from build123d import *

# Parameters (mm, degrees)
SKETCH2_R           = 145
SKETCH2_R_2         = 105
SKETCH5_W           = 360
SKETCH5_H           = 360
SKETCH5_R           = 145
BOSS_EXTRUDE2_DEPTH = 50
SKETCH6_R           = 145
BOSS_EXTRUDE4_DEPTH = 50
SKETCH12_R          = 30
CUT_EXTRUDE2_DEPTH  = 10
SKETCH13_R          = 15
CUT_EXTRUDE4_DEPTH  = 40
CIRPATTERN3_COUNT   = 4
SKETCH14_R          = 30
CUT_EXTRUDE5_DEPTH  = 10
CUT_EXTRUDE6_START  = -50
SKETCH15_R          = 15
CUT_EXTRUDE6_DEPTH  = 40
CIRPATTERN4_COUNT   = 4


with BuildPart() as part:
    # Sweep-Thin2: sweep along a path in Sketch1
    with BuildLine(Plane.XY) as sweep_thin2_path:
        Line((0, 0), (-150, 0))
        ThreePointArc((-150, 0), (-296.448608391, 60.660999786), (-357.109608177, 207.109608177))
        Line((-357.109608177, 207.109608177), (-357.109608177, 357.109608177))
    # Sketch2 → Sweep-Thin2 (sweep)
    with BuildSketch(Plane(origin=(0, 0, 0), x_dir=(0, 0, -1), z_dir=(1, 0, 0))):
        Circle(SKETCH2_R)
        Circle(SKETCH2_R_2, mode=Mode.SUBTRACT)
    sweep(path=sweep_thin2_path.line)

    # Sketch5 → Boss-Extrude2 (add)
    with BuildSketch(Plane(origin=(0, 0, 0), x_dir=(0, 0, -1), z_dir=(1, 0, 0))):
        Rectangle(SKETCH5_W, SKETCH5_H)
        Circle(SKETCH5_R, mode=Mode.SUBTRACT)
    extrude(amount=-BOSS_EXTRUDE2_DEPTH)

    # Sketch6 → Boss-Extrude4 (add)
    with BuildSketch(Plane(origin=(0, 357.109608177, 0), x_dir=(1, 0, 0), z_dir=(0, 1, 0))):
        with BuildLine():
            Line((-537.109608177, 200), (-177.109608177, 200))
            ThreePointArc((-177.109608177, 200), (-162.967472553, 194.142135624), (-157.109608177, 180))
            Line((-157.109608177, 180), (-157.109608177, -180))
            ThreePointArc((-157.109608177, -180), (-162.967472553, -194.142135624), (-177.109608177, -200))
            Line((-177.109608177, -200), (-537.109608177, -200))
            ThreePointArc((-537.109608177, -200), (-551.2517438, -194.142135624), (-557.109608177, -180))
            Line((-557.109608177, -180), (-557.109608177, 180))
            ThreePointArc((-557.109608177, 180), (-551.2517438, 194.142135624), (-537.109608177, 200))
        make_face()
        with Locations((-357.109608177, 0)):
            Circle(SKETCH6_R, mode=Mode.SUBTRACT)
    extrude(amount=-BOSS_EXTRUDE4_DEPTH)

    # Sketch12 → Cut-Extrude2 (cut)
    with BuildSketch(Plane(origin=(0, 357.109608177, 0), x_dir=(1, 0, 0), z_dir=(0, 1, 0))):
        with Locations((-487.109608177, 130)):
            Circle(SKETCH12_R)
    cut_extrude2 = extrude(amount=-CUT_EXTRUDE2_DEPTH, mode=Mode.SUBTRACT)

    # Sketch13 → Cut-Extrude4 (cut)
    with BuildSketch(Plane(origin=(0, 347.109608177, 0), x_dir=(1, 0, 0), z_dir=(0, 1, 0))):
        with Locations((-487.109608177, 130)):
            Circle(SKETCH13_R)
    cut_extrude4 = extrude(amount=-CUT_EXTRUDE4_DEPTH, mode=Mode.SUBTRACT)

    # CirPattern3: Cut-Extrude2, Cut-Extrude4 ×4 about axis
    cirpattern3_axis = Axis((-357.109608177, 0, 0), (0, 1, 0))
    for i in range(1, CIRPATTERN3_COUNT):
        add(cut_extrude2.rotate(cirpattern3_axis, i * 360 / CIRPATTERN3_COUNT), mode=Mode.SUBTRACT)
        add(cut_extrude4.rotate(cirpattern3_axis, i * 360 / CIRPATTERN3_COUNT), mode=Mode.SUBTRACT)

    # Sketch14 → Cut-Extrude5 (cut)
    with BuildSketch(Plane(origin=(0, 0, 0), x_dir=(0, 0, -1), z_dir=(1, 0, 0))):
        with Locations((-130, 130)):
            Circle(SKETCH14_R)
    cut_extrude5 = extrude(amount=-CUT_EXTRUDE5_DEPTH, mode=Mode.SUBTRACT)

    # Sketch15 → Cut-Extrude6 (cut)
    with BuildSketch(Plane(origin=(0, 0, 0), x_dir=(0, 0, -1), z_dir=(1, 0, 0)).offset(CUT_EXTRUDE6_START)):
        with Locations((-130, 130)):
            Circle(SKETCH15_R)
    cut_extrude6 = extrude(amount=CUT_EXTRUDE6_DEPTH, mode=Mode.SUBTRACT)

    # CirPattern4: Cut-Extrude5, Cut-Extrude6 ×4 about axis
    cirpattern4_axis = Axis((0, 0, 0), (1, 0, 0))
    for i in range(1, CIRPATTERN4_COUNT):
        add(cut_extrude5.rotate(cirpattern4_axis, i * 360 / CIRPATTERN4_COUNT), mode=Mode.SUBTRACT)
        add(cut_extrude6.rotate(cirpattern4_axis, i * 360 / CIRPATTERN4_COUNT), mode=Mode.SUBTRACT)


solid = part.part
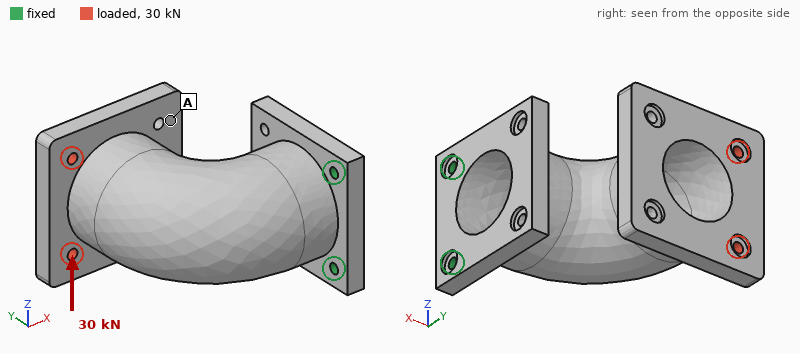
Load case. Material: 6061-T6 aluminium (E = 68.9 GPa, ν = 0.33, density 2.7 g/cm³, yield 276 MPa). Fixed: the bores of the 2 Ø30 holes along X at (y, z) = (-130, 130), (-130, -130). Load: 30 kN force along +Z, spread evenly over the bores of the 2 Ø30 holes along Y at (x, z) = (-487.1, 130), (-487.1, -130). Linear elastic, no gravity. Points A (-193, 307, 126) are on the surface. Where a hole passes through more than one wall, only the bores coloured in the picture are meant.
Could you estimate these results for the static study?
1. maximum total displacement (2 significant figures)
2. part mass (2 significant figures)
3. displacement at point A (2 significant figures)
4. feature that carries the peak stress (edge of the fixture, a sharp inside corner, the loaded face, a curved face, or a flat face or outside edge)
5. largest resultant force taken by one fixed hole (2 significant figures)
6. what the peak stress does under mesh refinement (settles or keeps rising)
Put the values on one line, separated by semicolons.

0.61 mm; 73 kg; 0.29 mm; edge of the fixture; 76 kN; keeps rising
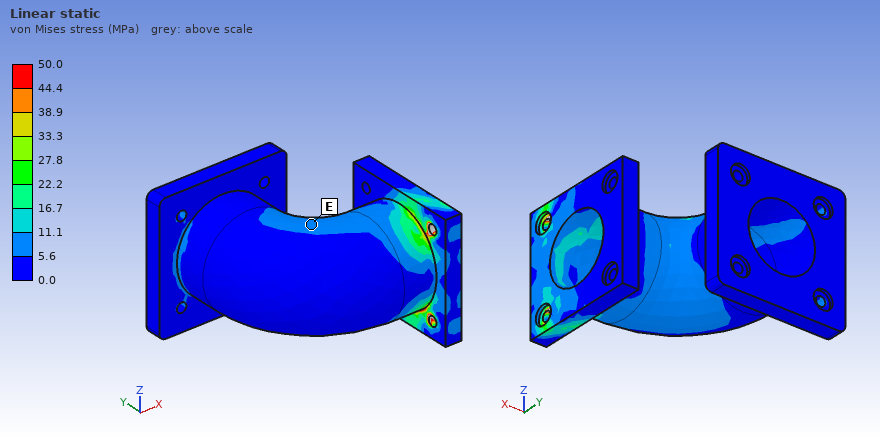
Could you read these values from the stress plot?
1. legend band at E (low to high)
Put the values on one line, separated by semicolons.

5.6 to 11.1 MPa
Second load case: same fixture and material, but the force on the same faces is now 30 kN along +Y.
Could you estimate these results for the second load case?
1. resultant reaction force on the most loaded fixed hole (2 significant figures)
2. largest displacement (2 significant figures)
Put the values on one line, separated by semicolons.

15 kN; 3.9 mm
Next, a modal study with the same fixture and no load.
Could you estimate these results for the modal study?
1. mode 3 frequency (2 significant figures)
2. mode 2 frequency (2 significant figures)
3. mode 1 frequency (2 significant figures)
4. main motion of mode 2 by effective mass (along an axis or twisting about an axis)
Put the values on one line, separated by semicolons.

530 Hz; 240 Hz; 75 Hz; along Z
